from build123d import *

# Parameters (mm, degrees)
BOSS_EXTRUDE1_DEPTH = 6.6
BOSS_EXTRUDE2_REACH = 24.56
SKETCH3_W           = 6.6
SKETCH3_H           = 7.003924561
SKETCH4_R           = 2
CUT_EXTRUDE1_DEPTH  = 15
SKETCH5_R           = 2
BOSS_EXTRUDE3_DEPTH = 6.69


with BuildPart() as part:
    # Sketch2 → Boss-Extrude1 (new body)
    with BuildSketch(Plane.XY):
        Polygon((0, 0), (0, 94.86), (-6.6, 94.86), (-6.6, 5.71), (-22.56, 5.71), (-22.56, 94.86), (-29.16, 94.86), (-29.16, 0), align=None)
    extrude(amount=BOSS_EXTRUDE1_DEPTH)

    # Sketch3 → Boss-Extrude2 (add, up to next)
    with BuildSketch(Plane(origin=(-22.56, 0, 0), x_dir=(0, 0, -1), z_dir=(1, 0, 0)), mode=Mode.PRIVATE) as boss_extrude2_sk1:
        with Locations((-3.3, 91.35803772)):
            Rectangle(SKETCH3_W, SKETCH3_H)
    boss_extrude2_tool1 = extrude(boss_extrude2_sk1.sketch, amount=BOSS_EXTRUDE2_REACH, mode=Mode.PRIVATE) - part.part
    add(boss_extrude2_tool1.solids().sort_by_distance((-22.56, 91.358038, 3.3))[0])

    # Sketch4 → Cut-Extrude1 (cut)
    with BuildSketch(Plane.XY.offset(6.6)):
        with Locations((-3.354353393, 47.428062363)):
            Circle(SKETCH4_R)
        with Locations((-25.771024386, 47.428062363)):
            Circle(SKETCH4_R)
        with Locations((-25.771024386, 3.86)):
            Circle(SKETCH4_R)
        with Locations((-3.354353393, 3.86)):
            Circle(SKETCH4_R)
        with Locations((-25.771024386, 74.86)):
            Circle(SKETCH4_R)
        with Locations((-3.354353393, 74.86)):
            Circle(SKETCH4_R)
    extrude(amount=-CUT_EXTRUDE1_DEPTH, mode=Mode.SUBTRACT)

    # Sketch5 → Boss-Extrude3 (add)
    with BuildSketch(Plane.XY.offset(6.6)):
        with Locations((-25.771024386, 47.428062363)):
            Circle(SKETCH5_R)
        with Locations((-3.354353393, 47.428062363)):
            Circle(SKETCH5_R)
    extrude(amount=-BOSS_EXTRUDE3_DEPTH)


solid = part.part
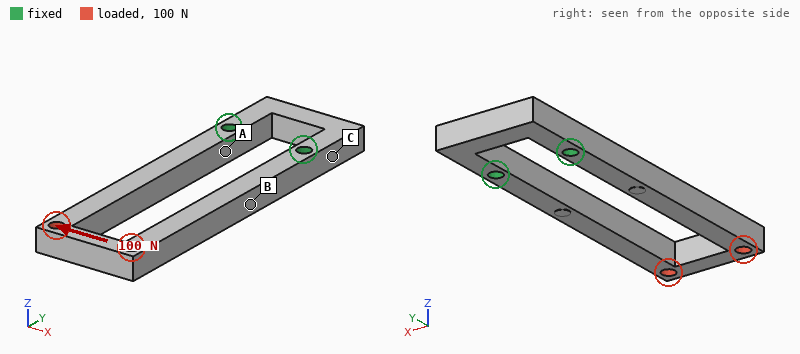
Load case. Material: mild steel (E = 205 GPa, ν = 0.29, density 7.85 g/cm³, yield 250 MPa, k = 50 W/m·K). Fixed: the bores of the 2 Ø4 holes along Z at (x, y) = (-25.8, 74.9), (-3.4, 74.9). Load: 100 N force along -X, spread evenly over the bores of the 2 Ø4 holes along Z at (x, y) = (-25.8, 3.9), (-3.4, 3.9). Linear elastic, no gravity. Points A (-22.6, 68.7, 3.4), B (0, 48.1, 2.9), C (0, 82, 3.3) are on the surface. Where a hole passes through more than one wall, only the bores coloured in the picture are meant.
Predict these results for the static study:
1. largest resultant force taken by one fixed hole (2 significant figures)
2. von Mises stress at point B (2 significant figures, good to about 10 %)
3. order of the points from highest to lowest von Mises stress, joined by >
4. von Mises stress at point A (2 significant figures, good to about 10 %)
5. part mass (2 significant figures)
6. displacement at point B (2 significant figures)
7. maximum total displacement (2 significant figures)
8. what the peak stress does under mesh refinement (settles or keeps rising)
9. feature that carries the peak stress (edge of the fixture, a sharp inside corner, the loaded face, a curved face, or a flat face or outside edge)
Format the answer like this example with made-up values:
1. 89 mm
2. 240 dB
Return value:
1. 150 N
2. 18 MPa
3. A > B > C
4. 33 MPa
5. 73 g
6. 18 µm
7. 67 µm
8. keeps rising
9. a sharp inside corner
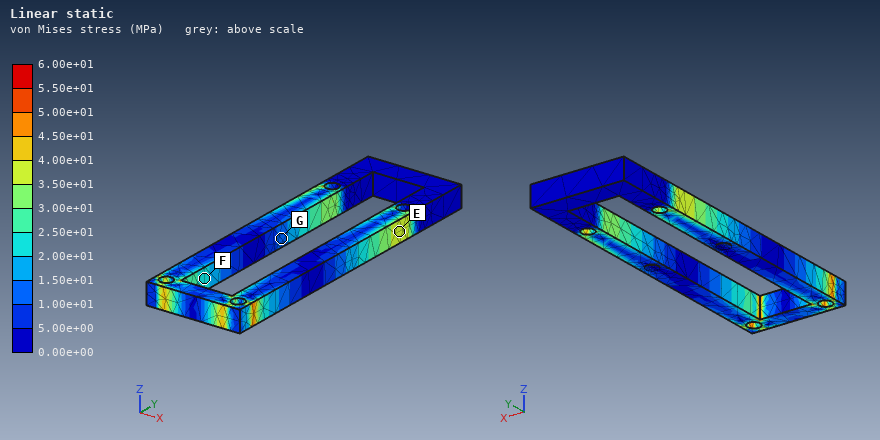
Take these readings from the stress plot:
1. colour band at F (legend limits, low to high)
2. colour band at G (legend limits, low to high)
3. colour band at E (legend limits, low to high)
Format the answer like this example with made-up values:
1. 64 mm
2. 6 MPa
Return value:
1. 2.00e+01 to 2.50e+01 MPa
2. 1.00e+01 to 1.50e+01 MPa
3. 3.50e+01 to 4.00e+01 MPa
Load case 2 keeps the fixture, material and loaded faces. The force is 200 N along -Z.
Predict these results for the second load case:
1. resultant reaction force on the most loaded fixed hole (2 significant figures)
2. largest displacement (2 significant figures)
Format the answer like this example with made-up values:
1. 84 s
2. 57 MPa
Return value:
1. 100 N
2. 0.38 mm
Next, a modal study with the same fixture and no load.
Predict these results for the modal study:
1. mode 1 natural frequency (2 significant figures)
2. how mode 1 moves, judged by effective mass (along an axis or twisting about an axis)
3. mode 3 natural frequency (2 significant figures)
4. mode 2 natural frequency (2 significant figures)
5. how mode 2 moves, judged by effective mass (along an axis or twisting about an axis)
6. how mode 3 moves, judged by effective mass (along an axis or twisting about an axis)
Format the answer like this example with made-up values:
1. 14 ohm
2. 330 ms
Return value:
1. 900 Hz
2. along Z
3. 2800 Hz
4. 1300 Hz
5. along X
6. twisting about Y
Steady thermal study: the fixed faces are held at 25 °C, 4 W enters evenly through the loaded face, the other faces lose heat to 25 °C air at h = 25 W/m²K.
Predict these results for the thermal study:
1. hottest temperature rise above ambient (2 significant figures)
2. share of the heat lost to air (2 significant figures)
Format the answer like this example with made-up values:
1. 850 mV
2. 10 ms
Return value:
1. 40 K
2. 53 %
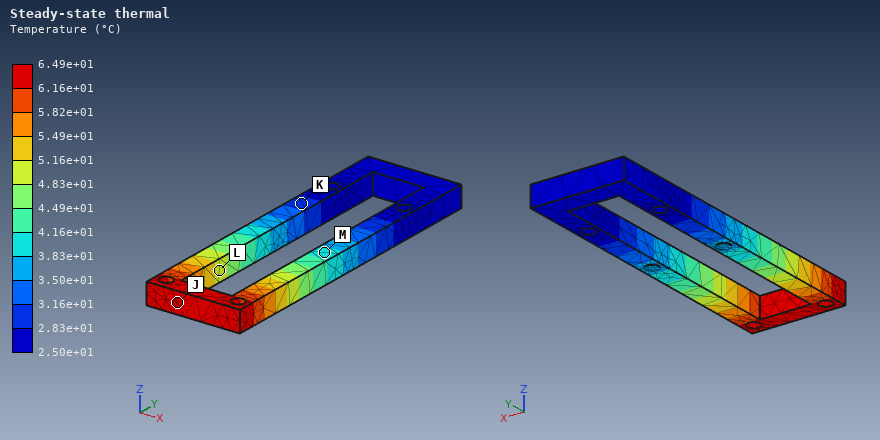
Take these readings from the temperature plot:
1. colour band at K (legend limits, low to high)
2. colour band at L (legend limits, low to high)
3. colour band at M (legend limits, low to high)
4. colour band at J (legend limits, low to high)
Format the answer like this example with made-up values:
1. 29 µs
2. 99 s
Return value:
1. 2.83e+01 to 3.16e+01 °C
2. 4.83e+01 to 5.16e+01 °C
3. 3.83e+01 to 4.16e+01 °C
4. 6.16e+01 to 6.49e+01 °C
